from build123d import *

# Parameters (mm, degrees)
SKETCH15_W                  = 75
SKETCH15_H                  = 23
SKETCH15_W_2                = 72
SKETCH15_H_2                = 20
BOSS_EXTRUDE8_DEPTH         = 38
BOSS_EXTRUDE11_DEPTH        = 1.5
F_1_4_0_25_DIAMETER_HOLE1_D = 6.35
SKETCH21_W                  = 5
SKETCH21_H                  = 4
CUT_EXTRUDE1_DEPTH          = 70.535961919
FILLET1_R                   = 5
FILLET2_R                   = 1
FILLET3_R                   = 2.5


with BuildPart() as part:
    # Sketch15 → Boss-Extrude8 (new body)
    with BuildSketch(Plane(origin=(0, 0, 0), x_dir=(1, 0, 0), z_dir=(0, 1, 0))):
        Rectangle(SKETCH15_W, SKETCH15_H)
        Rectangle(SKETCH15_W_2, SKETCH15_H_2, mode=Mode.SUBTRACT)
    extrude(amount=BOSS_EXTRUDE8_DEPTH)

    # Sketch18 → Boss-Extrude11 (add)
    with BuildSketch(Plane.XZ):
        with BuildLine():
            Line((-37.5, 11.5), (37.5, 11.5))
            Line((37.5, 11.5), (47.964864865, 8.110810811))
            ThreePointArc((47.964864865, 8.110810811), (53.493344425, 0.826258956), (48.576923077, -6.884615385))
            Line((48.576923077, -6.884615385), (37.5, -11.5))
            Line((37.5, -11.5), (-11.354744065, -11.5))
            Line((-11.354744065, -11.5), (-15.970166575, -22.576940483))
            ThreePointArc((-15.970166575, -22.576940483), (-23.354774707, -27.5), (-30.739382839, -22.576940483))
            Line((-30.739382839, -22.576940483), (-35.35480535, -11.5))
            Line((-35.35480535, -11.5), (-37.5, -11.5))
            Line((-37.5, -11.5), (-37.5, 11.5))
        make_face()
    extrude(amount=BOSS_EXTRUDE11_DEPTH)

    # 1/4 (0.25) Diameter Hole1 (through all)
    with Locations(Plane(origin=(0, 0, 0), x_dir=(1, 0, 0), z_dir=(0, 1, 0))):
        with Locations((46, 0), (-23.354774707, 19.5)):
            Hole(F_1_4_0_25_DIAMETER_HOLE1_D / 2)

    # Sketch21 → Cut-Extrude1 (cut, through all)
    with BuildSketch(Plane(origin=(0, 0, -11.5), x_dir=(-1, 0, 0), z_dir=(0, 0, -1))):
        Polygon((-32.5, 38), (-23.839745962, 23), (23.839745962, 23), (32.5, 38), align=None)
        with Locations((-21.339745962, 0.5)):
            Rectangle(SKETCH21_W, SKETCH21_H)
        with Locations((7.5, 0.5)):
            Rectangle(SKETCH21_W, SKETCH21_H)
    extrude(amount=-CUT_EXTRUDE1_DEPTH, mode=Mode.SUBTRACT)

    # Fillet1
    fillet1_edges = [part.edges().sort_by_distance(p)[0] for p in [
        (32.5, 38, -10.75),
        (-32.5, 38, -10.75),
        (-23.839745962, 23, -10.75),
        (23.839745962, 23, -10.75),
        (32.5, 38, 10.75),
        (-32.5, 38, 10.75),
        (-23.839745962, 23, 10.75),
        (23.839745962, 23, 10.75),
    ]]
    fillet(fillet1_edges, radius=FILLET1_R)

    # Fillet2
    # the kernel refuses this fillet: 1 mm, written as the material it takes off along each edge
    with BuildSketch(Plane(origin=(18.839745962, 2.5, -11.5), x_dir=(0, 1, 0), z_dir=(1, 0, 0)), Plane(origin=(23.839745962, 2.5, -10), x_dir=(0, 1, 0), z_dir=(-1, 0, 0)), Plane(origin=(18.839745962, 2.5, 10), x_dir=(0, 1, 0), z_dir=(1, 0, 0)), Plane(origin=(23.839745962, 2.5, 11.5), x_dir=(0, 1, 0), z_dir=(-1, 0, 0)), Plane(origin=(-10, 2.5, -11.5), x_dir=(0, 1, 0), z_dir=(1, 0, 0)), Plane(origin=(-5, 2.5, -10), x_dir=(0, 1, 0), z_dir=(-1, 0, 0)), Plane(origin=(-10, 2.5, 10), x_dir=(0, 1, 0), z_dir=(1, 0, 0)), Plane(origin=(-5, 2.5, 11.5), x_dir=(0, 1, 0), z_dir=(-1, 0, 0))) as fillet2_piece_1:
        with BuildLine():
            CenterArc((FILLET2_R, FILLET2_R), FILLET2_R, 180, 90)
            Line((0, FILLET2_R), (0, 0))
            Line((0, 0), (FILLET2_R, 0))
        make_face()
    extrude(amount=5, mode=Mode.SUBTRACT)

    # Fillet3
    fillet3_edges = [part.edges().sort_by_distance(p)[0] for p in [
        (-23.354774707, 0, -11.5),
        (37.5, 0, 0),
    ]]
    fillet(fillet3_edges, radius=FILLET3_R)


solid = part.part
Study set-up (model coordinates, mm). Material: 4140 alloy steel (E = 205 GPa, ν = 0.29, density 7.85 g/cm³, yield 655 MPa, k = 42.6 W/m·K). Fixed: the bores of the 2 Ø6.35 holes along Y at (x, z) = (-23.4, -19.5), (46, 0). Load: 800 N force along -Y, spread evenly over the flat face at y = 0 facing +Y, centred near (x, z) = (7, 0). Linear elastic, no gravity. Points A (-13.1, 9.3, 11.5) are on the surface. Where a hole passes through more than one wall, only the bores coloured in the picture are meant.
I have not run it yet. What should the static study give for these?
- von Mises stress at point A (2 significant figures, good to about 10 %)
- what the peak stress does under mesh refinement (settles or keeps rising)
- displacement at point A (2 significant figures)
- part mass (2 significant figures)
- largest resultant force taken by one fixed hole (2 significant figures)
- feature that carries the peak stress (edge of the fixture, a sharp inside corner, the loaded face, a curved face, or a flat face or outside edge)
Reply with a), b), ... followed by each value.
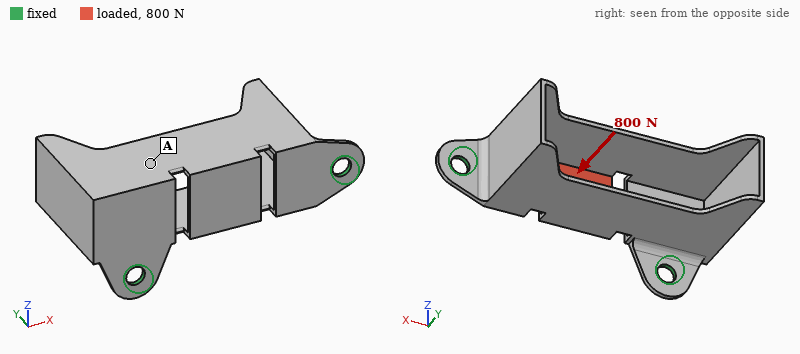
a) 53 MPa
b) keeps rising
c) 0.34 mm
d) 88 g
e) 460 N
f) edge of the fixture
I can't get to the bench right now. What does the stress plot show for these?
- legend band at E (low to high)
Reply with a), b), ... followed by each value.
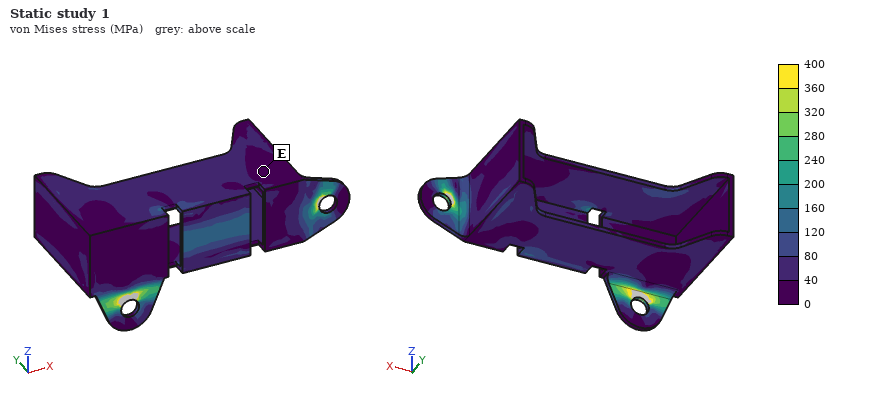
a) 0 to 40 MPa
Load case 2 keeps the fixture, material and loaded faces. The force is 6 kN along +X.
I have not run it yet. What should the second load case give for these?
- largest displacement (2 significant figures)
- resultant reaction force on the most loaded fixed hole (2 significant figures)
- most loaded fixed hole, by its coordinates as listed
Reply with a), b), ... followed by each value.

a) 0.12 mm
b) 4.2 kN
c) (46, 0)
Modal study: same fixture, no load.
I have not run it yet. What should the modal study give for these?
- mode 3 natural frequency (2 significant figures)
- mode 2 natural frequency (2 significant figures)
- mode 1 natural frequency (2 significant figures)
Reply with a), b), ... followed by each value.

a) 2500 Hz
b) 1400 Hz
c) 590 Hz
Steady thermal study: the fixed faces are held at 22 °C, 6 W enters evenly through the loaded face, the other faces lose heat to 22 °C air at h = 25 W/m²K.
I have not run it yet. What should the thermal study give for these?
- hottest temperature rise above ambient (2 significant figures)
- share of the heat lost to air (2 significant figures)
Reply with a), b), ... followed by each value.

a) 44 K
b) 70 %
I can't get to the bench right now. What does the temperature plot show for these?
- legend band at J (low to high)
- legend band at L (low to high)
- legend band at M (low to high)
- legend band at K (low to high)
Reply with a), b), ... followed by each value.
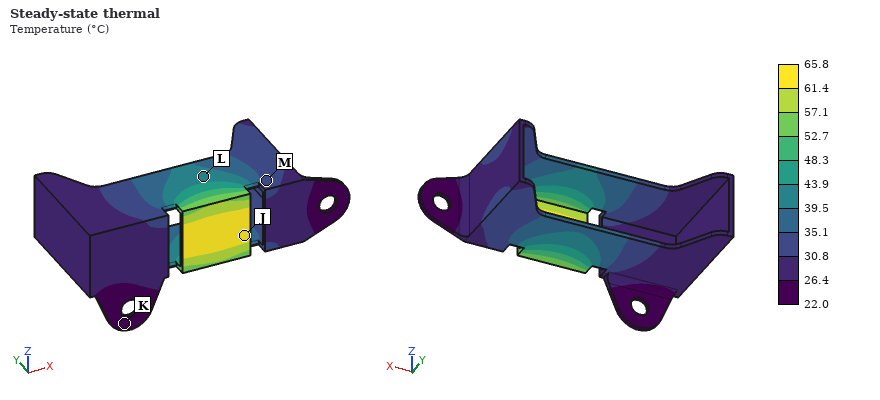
a) 61.4 to 65.8 °C
b) 39.5 to 43.9 °C
c) 30.8 to 35.1 °C
d) 22.0 to 26.4 °C
